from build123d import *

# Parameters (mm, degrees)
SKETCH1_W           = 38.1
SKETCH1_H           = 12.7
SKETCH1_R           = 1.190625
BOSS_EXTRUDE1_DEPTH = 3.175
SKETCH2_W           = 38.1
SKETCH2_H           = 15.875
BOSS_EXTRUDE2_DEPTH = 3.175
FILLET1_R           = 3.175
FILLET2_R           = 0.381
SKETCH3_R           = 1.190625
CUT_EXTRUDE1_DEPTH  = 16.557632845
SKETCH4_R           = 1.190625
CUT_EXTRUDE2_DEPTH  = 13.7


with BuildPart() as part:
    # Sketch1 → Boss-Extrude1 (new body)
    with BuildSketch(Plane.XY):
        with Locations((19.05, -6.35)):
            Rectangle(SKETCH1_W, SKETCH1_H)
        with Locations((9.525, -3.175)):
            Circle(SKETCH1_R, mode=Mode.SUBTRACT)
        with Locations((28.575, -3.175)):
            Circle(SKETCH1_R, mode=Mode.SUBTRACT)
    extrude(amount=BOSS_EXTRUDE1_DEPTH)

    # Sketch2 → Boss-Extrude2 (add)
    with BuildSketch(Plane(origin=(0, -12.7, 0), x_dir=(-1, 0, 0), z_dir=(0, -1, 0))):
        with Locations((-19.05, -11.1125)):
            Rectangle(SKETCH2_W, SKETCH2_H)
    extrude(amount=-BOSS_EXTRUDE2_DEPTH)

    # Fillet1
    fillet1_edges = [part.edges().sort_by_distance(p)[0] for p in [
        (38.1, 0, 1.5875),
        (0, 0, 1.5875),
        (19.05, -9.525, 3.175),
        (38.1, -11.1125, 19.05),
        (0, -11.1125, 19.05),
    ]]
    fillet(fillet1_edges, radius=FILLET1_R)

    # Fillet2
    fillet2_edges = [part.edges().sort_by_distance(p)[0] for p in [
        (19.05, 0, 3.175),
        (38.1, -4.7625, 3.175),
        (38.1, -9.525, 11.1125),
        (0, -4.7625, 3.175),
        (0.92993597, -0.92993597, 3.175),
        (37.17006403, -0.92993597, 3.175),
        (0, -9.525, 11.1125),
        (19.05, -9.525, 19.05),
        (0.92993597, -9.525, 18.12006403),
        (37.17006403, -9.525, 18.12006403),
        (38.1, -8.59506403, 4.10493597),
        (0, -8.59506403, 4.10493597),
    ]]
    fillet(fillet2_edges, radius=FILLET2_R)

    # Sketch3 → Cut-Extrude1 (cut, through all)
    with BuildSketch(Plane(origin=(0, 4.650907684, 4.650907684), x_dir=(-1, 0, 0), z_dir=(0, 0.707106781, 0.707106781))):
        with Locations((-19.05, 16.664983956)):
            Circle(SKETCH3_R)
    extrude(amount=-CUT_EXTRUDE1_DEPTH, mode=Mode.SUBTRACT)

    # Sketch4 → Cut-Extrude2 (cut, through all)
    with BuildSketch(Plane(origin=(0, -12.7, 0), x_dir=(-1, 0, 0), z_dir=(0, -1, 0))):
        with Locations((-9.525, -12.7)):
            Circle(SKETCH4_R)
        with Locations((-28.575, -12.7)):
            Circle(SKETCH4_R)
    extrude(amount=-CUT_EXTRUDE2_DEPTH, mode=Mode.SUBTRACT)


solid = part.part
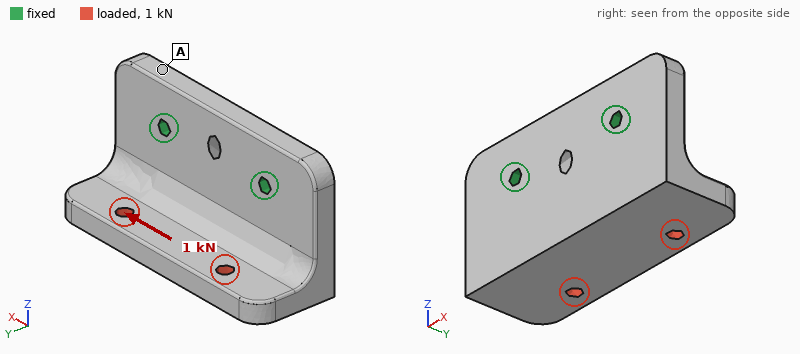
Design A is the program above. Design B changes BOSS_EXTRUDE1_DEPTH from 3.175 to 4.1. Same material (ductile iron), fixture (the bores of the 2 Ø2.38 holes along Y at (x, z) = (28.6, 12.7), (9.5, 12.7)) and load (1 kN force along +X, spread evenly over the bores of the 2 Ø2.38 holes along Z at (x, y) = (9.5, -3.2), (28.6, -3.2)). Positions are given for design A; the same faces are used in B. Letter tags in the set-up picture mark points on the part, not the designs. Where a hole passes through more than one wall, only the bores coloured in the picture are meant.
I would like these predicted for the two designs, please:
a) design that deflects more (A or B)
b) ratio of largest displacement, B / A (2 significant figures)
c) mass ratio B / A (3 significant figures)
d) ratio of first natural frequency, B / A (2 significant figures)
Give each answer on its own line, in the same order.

A
0.77
1.09
0.95
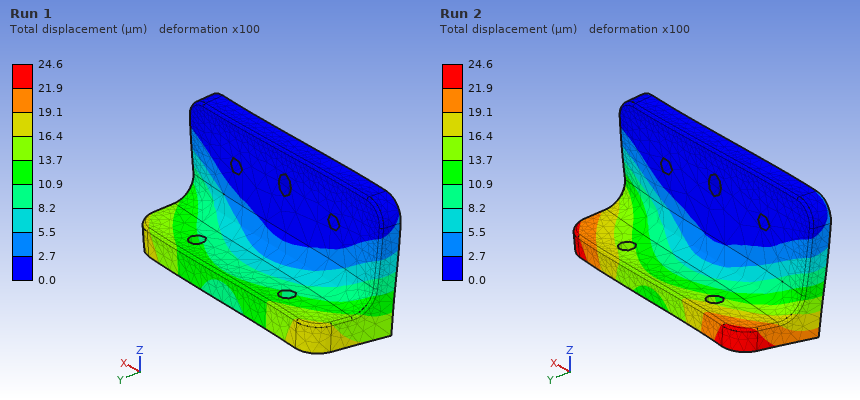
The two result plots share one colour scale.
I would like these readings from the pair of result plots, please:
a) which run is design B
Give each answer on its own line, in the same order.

Run 1
